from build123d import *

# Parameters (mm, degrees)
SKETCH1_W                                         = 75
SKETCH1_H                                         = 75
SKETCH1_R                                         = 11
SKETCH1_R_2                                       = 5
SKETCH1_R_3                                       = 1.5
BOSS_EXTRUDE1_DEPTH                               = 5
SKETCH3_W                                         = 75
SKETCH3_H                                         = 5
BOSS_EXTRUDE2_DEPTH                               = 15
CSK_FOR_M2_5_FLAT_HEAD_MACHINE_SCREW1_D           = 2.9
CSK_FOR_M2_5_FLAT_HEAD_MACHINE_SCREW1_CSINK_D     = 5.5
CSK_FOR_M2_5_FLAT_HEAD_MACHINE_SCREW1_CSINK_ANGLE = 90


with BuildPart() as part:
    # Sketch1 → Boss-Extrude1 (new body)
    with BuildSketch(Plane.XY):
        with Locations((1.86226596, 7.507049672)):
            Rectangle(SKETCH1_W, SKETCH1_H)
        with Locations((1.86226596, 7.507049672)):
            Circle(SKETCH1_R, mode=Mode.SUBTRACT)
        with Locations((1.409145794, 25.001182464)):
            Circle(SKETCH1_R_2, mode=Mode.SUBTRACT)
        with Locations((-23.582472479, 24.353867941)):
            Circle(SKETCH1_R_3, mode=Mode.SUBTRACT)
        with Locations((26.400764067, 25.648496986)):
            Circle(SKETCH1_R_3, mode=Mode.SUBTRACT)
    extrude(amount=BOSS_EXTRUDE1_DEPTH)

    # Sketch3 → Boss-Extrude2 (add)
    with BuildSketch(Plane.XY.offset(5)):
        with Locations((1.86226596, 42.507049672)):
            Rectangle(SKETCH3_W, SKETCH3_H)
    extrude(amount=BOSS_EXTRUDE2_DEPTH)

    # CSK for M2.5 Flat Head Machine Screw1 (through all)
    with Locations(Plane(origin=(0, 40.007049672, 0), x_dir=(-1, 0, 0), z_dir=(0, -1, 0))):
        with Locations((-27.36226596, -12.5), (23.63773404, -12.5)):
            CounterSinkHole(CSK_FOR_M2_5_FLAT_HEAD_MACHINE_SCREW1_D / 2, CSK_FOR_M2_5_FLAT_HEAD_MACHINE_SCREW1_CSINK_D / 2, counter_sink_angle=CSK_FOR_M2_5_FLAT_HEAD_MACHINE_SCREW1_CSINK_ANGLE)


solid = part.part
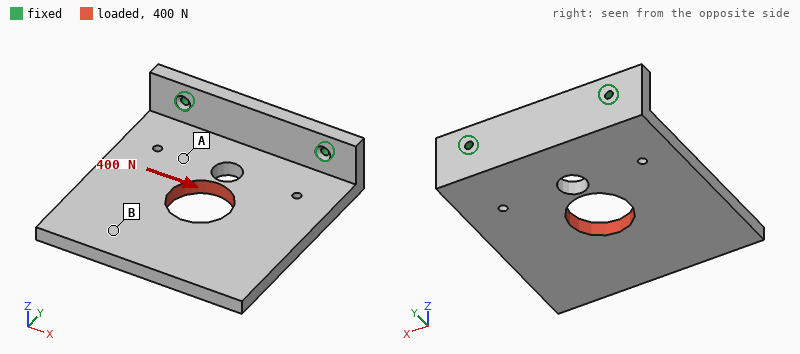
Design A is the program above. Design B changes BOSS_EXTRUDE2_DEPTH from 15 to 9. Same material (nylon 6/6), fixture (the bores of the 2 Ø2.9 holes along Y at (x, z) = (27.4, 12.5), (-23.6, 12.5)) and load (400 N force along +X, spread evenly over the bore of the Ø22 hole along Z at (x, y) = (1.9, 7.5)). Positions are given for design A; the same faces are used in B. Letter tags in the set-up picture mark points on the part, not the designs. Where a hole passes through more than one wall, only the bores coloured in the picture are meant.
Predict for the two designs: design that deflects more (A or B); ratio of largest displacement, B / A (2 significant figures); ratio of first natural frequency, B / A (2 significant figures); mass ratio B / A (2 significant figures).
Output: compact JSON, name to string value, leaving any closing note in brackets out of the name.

{"design that deflects more": "B", "ratio of largest displacement, B / A": "1.1", "ratio of first natural frequency, B / A": "0.88", "mass ratio B / A": "0.93"}
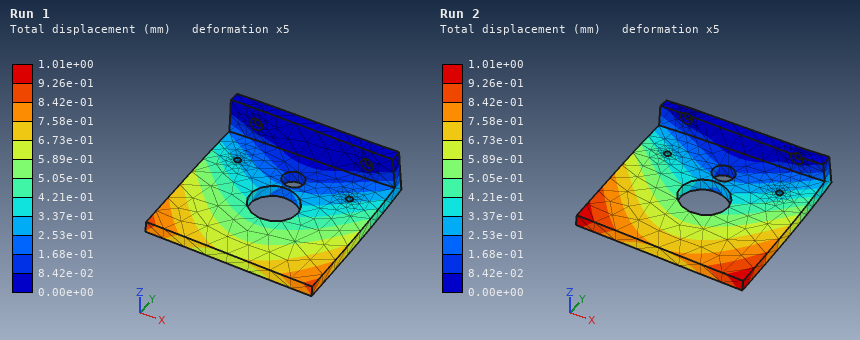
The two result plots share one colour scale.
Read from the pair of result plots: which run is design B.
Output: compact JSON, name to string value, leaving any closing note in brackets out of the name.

{"which run is design B": "Run 2"}
